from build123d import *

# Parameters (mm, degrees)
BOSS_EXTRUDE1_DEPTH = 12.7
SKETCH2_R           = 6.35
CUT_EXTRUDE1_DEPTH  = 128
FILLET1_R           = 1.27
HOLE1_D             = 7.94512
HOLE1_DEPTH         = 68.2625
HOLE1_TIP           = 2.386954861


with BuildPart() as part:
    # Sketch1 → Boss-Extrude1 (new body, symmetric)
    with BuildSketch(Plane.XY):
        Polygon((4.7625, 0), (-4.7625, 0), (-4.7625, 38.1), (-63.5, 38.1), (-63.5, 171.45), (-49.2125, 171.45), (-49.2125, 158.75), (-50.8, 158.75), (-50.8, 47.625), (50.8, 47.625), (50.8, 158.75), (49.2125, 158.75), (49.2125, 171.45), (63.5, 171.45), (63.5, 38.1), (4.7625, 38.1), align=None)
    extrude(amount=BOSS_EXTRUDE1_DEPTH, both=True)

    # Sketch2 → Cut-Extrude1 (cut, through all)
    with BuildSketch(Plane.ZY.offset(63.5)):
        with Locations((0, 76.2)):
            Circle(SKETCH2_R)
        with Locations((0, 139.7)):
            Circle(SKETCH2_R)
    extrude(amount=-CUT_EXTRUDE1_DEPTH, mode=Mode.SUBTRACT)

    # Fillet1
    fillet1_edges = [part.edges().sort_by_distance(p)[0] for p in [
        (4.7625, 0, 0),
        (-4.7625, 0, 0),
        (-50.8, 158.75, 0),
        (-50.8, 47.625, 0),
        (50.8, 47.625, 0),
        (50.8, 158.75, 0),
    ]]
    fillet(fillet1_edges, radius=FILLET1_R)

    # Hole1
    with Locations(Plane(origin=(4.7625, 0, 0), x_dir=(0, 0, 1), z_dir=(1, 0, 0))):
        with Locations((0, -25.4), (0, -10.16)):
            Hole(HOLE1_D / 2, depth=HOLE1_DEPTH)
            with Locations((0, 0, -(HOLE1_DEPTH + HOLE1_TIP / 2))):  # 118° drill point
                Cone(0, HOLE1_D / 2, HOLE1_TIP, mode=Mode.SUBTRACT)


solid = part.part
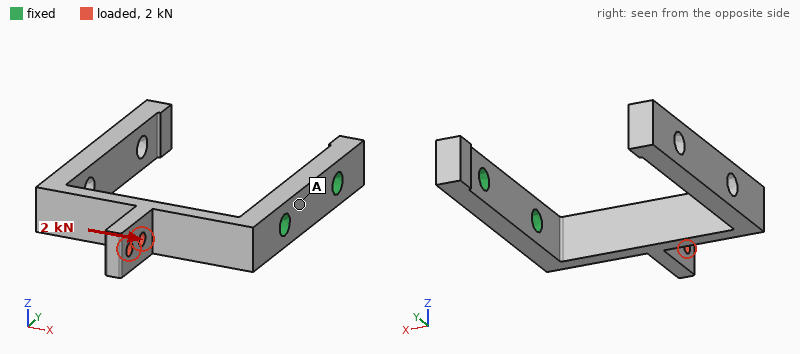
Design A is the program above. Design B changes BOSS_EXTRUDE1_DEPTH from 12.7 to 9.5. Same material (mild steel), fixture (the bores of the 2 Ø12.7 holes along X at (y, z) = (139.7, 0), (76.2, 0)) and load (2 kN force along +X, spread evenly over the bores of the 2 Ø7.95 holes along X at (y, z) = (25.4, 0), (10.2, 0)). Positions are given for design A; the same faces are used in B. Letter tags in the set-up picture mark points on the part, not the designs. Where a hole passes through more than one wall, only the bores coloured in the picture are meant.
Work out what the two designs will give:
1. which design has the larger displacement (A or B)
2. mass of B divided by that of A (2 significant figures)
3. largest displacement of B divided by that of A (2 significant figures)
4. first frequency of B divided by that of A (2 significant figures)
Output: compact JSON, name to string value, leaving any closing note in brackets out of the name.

{"which design has the larger displacement": "B", "mass of B divided by that of A": "0.73", "largest displacement of B divided by that of A": "1.3", "first frequency of B divided by that of A": "1.0"}
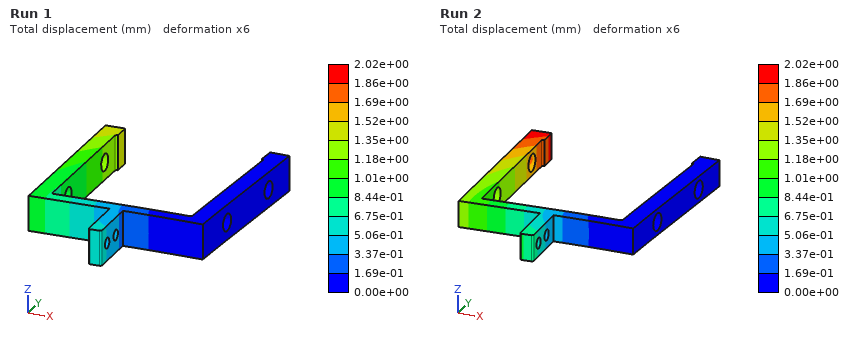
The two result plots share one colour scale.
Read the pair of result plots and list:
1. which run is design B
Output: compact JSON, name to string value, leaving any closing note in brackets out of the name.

{"which run is design B": "Run 2"}
